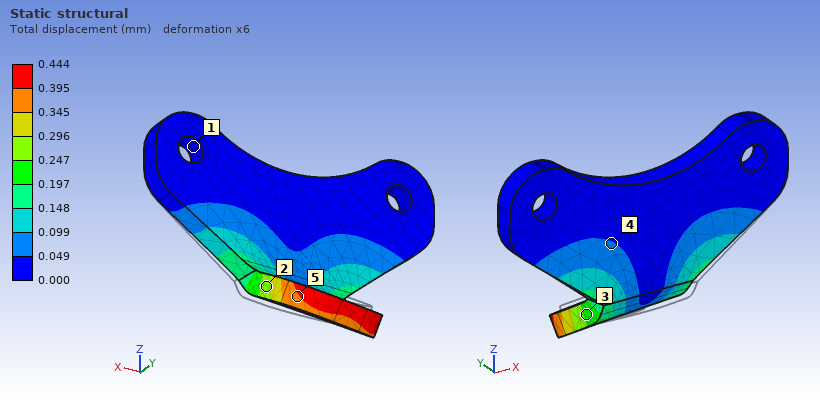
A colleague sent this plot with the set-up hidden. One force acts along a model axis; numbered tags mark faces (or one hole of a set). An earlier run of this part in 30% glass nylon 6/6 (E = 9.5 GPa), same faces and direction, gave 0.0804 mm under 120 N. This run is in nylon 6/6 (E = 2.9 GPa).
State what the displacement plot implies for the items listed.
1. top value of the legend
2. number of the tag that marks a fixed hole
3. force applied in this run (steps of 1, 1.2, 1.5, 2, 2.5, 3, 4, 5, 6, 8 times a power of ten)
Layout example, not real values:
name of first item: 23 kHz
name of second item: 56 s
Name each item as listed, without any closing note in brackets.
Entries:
top value of the legend: 0.444 mm
number of the tag that marks a fixed hole: 1
force applied in this run: 200 N
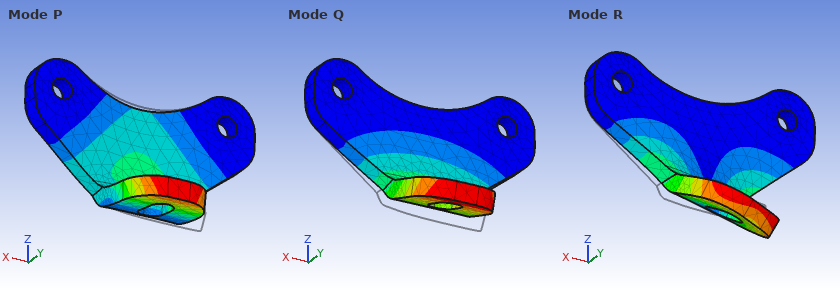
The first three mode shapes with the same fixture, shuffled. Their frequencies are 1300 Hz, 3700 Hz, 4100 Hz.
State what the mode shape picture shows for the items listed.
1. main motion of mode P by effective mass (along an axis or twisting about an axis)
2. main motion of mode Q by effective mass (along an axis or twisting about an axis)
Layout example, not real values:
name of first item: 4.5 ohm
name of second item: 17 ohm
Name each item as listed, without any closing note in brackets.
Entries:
main motion of mode P by effective mass: along Y
main motion of mode Q by effective mass: along Y
